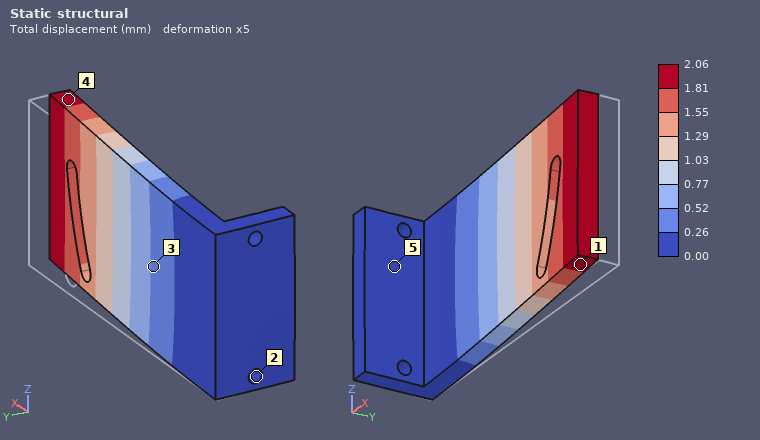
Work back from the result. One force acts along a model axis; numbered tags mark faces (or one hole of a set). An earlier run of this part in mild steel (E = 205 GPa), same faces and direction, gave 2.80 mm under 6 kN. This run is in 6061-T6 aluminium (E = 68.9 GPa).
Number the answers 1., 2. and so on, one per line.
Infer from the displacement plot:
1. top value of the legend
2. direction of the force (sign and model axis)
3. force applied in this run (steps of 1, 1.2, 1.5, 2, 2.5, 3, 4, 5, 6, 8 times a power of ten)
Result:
1. 2.06 mm
2. -Y
3. 1.5 kN
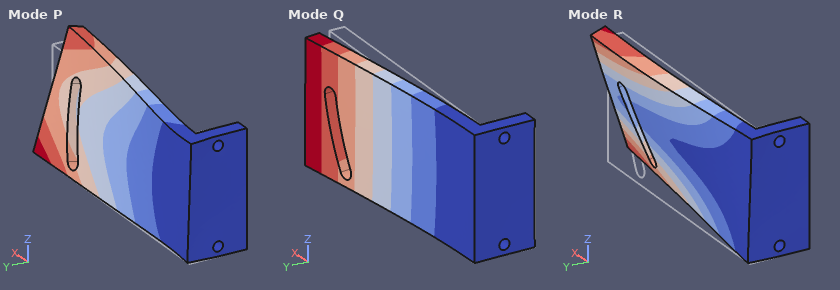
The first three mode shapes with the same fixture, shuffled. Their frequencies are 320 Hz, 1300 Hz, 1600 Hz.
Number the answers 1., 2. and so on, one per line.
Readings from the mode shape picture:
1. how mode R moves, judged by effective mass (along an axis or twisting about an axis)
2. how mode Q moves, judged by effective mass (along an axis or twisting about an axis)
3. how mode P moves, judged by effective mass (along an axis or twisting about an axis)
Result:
1. along Z
2. along Y
3. along Z
